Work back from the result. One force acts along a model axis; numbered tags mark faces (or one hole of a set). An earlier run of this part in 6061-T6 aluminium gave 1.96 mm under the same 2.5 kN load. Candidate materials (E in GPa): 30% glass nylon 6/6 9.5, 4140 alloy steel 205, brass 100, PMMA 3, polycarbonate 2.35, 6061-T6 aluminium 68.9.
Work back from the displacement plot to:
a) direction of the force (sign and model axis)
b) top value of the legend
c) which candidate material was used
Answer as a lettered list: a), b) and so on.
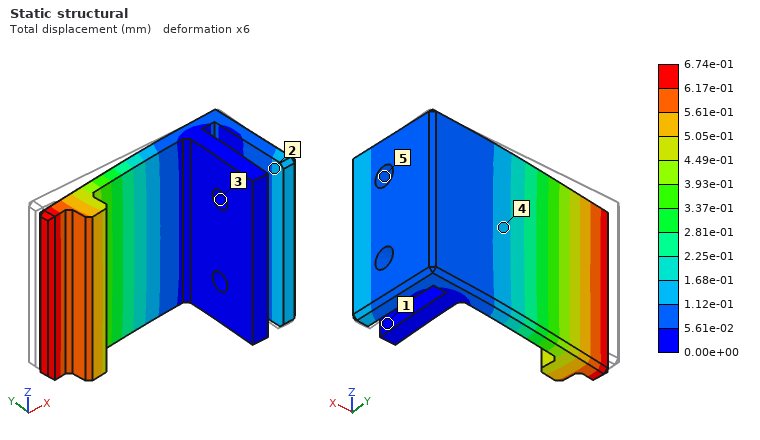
a) -Y
b) 6.74e-01 mm
c) 4140 alloy steel
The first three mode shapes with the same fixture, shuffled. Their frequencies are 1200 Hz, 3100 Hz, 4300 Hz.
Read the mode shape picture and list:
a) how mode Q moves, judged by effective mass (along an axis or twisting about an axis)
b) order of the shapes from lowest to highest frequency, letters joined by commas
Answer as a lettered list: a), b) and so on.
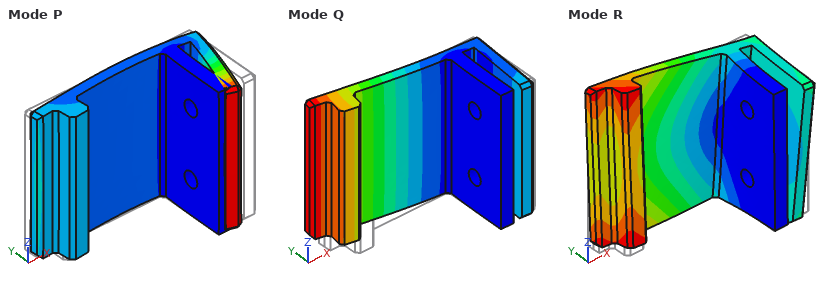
a) along Y
b) Q, R, P
